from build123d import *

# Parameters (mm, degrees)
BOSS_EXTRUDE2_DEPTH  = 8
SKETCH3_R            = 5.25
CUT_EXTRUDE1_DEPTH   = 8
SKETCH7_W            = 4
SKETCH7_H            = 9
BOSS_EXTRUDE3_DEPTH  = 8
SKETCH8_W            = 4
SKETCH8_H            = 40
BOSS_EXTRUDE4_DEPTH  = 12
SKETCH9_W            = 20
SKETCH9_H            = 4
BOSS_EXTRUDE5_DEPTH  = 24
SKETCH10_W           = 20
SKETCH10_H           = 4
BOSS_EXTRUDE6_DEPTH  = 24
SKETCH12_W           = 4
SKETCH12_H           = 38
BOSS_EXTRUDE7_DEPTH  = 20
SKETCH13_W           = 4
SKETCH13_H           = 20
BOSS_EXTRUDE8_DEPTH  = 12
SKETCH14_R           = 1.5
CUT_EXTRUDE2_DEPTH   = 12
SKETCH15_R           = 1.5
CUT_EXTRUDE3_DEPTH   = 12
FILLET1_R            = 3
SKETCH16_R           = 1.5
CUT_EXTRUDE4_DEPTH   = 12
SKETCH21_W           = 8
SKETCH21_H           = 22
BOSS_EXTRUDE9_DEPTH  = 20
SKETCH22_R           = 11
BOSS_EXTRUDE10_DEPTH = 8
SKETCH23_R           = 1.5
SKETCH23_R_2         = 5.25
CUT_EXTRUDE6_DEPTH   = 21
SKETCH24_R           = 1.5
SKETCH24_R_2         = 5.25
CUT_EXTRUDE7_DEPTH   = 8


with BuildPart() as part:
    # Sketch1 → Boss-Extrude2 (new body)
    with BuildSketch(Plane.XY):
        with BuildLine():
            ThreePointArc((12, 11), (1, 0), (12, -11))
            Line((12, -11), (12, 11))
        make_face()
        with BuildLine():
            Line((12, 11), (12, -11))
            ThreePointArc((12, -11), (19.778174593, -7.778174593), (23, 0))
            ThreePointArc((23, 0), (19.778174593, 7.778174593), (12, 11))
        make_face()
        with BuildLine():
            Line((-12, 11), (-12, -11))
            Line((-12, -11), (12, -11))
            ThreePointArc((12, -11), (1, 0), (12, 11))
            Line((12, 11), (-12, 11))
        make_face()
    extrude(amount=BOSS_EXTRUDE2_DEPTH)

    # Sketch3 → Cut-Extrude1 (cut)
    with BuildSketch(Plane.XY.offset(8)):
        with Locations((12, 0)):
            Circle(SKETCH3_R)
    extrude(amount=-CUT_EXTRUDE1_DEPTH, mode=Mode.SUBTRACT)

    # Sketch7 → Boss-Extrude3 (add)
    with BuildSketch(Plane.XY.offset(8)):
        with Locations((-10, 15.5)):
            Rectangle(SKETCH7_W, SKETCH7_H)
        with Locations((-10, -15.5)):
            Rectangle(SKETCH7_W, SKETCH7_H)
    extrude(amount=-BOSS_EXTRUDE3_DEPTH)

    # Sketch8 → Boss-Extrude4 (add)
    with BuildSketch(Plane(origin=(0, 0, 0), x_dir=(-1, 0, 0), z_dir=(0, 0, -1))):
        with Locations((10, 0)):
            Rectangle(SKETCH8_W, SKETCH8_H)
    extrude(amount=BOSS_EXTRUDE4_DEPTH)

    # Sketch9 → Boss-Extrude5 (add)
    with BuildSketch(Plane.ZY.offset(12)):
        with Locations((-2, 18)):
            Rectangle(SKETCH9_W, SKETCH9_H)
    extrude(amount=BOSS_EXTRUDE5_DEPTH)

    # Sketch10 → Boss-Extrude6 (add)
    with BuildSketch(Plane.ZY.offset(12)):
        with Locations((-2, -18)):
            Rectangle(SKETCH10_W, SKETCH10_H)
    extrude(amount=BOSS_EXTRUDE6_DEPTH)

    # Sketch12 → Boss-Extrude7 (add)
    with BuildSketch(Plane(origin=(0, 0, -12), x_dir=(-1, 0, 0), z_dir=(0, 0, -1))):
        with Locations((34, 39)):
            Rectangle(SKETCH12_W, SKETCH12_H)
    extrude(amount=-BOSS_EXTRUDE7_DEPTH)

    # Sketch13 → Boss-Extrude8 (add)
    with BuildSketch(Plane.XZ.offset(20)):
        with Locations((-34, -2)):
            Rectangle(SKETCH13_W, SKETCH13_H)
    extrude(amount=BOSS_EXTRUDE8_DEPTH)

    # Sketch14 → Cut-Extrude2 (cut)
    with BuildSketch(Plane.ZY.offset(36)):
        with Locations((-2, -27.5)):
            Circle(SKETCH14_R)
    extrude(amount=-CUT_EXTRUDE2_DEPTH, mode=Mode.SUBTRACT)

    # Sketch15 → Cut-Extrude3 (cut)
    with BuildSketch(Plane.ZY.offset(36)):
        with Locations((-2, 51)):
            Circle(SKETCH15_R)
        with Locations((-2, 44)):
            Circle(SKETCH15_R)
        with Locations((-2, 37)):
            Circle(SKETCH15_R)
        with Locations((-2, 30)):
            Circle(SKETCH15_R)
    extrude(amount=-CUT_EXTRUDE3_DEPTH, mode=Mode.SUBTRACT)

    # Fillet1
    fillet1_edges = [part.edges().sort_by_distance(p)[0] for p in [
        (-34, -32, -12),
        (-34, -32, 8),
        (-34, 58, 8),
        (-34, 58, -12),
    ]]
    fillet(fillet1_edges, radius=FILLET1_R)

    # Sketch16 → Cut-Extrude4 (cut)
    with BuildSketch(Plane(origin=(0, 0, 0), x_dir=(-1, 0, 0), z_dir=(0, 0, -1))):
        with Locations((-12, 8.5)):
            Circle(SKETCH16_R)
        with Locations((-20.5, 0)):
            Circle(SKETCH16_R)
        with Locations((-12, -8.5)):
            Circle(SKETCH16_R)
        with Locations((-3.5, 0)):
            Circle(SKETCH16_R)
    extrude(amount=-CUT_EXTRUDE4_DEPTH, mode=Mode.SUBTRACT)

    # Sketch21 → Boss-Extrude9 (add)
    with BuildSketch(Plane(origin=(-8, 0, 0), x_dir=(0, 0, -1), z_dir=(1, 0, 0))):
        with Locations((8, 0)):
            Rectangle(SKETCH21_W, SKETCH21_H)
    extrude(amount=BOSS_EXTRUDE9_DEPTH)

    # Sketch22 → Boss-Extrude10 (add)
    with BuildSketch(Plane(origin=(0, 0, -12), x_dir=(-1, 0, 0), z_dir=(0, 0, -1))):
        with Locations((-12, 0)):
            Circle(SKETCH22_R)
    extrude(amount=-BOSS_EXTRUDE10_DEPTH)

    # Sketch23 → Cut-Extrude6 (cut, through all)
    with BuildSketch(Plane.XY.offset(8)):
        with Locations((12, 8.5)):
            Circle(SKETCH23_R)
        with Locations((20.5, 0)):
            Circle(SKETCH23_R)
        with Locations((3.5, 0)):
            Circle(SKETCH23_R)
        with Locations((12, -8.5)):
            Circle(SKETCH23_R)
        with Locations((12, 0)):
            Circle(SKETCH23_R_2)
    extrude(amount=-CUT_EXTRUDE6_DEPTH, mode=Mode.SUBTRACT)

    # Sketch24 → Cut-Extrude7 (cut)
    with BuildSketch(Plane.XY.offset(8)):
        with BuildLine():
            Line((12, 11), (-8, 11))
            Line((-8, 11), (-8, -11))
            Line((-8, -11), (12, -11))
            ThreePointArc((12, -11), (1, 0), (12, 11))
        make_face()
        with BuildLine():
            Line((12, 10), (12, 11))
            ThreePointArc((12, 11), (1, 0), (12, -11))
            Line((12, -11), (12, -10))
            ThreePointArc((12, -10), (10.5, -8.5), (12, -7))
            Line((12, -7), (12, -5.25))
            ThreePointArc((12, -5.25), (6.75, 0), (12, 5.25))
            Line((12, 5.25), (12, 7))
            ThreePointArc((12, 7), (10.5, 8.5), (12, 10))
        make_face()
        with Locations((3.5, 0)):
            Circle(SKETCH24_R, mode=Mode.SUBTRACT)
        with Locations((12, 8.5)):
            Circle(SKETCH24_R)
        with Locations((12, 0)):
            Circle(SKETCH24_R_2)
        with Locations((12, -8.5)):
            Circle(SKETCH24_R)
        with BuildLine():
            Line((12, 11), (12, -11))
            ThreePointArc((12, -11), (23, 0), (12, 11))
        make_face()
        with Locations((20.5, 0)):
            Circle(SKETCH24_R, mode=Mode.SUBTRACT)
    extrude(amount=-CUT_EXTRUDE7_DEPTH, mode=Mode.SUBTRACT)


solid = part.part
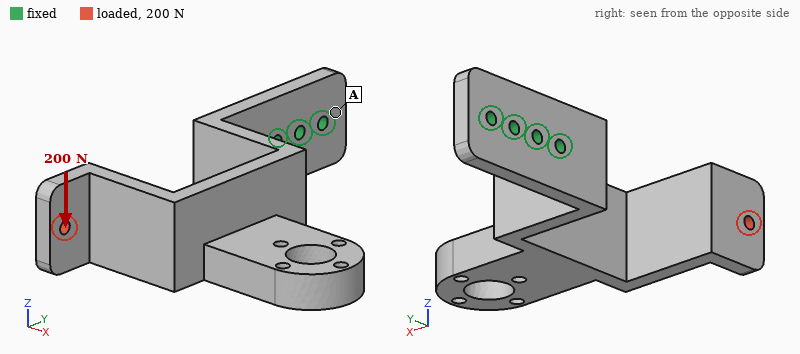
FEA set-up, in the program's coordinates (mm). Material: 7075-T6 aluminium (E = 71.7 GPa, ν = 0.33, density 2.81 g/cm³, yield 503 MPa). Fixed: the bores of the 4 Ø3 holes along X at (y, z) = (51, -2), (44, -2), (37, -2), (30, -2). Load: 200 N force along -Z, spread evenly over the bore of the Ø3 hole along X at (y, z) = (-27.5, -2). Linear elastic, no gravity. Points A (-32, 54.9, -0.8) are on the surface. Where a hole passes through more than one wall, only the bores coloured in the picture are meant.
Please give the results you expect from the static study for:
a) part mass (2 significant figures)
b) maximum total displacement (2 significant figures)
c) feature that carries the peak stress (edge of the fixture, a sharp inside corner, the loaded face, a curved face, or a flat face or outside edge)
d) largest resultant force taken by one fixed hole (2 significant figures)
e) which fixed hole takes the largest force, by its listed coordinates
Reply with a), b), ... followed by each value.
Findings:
a) 42 g
b) 1.3 mm
c) a flat face or outside edge
d) 830 N
e) (30, -2)
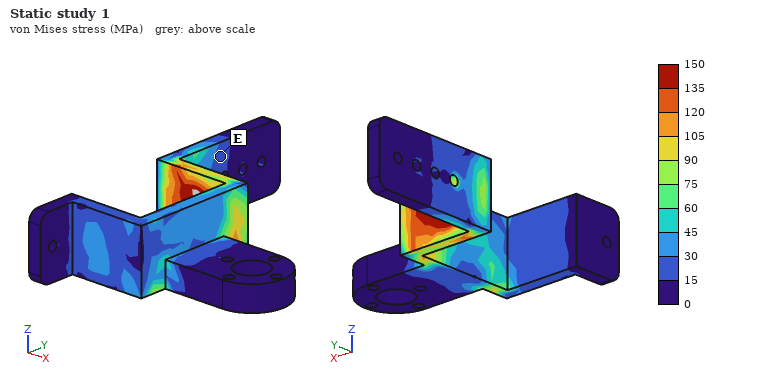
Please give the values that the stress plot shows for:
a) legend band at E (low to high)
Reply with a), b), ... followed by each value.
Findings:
a) 15 to 30 MPa
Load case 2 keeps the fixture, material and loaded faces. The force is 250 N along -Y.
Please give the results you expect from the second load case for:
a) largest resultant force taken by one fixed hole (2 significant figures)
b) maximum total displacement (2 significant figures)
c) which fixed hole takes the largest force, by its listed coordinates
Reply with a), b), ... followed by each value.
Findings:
a) 160 N
b) 1.2 mm
c) (30, -2)
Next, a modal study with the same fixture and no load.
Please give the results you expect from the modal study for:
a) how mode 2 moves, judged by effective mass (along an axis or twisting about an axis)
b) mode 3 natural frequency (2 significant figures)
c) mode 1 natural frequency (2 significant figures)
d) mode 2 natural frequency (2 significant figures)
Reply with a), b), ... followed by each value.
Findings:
a) along Z
b) 1100 Hz
c) 360 Hz
d) 720 Hz
